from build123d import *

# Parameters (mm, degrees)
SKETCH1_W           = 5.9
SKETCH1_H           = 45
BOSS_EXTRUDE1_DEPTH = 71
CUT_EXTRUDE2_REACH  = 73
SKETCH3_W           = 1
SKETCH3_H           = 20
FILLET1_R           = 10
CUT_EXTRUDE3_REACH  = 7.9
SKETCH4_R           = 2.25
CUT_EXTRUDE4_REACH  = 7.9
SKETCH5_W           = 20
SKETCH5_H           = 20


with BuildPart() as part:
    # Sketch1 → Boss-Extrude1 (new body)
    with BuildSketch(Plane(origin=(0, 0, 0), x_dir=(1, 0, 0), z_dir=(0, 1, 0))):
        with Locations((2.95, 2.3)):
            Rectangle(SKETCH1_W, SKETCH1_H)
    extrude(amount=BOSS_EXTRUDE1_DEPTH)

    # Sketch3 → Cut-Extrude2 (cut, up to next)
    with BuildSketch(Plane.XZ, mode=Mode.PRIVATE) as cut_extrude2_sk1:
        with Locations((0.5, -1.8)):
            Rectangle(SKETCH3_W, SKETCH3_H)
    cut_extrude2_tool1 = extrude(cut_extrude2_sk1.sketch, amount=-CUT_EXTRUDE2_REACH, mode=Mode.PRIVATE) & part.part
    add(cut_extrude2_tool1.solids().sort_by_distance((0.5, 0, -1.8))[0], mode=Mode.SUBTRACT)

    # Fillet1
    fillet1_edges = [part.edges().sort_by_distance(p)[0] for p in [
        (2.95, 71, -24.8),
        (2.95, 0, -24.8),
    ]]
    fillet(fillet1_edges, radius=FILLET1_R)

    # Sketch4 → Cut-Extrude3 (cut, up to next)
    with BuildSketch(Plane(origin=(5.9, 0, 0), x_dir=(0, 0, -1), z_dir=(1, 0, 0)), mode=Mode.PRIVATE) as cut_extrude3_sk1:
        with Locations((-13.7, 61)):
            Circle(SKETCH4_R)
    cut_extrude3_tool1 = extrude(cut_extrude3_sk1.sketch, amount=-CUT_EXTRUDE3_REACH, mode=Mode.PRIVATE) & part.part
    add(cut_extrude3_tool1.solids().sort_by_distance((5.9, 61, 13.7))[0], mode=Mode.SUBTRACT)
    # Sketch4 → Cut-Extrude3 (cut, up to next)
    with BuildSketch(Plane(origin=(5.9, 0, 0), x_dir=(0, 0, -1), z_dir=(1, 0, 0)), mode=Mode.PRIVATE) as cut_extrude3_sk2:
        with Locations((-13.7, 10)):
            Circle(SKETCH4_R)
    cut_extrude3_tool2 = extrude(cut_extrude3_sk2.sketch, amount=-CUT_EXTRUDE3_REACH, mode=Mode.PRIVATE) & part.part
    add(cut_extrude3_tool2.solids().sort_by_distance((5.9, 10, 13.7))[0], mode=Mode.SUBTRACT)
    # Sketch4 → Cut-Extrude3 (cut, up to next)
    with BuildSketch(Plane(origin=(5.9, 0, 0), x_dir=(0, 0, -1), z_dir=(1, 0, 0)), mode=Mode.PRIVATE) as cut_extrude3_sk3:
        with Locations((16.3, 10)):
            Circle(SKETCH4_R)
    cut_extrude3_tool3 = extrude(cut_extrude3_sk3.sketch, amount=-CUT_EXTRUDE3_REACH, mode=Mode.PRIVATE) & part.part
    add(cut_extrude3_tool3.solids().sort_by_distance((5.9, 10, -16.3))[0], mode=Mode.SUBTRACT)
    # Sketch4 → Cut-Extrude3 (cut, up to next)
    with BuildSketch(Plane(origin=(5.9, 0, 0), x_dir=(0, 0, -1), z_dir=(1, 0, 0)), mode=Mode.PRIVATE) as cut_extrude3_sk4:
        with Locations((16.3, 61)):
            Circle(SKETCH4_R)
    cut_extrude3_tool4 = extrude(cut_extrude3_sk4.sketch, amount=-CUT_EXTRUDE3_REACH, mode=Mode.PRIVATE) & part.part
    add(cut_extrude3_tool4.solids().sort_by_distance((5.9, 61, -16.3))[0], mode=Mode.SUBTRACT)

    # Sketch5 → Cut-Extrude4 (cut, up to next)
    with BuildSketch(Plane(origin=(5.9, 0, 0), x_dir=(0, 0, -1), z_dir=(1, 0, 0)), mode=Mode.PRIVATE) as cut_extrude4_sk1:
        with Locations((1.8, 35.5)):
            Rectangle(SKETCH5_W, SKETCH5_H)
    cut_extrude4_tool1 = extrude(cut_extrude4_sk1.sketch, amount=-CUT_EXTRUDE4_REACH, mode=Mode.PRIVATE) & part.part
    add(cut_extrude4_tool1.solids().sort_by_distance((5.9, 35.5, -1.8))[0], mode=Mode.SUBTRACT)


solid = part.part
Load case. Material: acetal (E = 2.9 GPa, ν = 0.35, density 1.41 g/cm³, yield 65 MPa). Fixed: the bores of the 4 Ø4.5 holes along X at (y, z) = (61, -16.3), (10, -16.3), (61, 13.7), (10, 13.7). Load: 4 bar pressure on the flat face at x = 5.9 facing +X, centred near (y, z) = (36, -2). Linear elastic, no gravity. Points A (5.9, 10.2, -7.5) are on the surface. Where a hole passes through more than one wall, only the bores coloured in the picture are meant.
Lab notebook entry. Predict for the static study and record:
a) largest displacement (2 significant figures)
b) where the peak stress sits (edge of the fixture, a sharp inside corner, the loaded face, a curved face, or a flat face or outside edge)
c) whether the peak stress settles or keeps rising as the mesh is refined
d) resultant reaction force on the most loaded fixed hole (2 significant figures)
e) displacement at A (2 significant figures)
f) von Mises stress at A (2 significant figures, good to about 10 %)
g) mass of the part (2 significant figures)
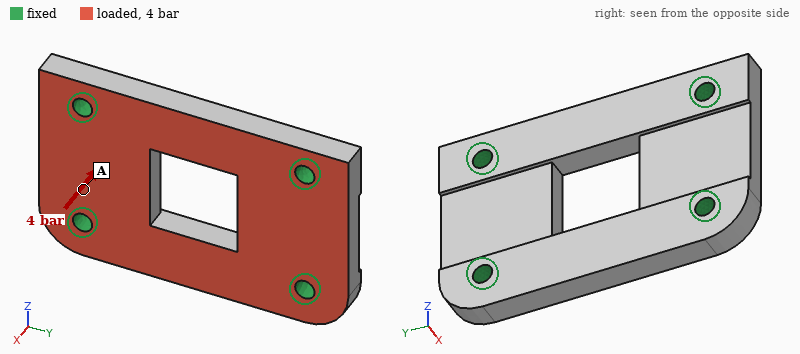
0.17 mm
edge of the fixture
keeps rising
280 N
0.028 mm
4.6 MPa
21 g
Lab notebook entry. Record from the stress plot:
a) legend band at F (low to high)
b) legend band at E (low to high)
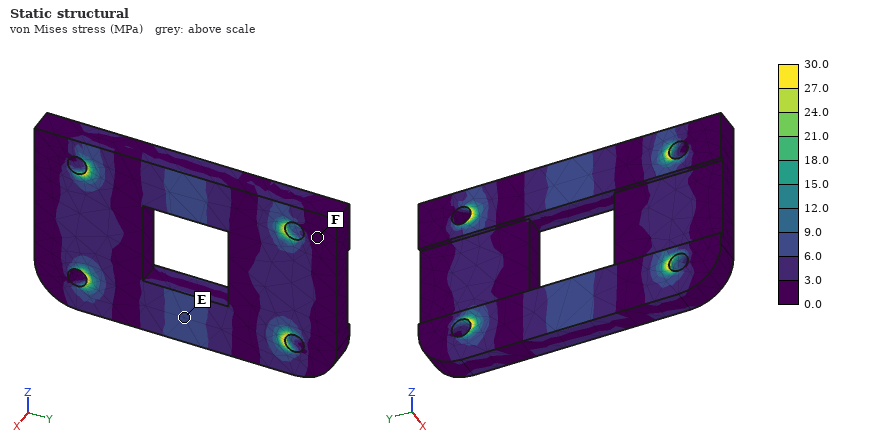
0.0 to 3.0 MPa
6.0 to 9.0 MPa
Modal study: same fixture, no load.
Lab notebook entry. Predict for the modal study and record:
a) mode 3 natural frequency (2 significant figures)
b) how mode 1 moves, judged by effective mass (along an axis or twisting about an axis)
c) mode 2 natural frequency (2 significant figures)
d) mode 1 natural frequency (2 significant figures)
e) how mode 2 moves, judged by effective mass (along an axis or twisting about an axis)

5600 Hz
along X
3600 Hz
3300 Hz
twisting about Y
